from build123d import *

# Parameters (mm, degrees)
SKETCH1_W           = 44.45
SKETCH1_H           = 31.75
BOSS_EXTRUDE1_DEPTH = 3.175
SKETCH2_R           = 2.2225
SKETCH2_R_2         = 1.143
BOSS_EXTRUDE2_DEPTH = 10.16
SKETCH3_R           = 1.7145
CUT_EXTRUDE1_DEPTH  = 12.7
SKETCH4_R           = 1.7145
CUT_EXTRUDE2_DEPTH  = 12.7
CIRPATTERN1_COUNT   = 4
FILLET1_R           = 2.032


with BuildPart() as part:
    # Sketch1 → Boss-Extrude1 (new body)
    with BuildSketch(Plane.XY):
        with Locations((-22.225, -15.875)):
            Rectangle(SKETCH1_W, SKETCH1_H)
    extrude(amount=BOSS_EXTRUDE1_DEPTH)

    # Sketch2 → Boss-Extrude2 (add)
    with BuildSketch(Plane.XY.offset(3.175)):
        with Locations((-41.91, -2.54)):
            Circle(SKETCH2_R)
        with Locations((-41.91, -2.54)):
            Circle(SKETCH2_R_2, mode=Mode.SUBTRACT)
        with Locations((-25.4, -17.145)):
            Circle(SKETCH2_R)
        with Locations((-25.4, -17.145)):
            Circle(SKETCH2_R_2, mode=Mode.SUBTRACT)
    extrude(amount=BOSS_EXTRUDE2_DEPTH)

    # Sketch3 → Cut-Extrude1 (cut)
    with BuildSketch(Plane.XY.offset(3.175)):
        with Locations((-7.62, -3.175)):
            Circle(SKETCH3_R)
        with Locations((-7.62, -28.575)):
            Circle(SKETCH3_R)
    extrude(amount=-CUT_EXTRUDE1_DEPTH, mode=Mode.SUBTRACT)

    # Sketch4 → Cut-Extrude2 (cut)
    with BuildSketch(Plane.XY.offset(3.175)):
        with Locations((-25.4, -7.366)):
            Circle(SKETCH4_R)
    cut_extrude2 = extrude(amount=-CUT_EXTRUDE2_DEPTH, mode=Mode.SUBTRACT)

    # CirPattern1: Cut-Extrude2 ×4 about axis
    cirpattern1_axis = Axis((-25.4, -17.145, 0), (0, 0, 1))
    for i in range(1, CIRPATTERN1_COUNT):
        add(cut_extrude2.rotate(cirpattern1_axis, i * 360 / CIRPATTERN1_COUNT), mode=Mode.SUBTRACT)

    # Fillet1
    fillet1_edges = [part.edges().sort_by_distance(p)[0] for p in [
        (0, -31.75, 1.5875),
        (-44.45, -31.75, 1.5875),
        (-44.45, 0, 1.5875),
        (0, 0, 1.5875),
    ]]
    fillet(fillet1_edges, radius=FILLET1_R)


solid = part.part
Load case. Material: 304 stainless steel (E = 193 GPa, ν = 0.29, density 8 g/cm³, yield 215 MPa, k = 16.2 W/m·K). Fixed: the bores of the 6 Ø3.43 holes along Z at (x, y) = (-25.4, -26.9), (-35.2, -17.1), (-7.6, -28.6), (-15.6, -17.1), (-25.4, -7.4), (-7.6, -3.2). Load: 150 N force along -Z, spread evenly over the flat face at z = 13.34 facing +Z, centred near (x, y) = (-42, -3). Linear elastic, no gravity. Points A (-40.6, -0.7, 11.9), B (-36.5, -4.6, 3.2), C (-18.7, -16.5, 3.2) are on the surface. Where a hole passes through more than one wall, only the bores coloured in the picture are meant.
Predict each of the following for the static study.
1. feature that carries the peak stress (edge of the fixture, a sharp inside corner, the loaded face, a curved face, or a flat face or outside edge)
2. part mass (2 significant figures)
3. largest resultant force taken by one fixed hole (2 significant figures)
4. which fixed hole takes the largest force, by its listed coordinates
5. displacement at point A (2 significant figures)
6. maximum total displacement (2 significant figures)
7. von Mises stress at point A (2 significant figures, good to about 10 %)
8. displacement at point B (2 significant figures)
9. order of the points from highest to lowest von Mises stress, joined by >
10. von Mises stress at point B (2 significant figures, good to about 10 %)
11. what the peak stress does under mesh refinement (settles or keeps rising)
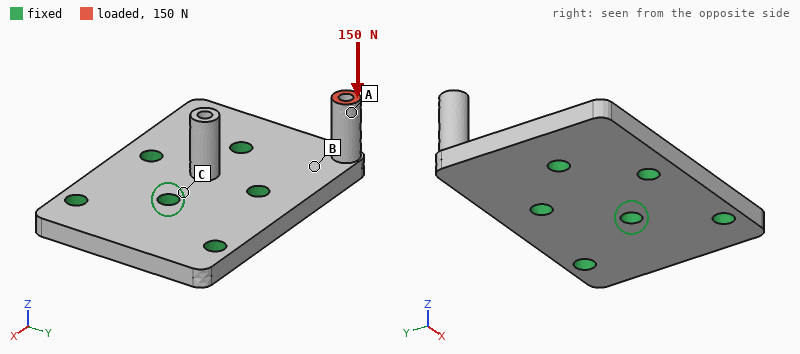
edge of the fixture
36 g
110 N
(-35.2, -17.1)
24 µm
28 µm
13 MPa
7.3 µm
B > A > C
35 MPa
keeps rising
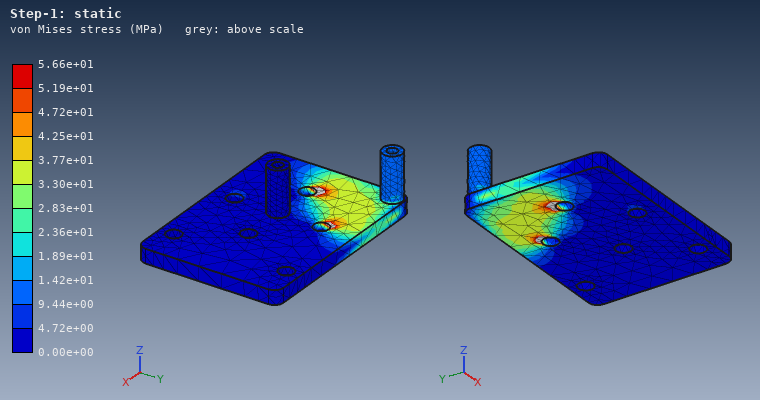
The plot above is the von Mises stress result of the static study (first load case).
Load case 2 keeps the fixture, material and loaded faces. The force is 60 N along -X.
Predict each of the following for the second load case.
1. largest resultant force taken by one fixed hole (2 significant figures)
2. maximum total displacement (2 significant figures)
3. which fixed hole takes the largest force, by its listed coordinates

58 N
23 µm
(-25.4, -7.4)
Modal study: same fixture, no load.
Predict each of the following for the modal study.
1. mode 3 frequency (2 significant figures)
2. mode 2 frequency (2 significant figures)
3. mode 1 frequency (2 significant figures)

16 kHz
16 kHz
9100 Hz
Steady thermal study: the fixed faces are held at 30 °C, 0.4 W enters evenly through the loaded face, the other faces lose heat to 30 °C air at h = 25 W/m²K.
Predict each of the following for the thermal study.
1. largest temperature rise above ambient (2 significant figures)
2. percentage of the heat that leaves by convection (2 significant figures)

26 K
31 %
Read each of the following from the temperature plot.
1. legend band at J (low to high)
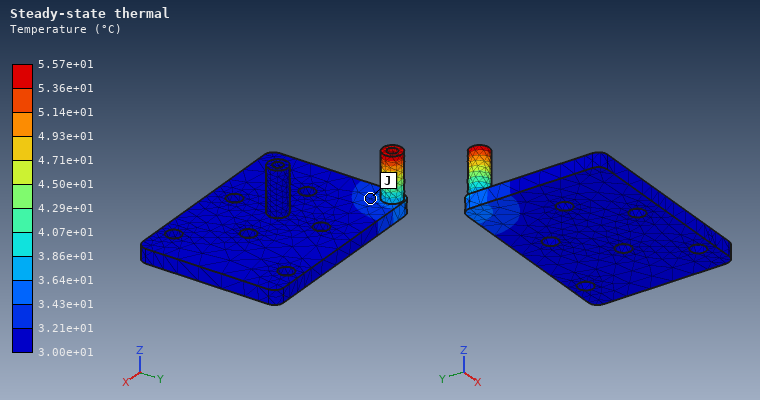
3.21e+01 to 3.43e+01 °C
